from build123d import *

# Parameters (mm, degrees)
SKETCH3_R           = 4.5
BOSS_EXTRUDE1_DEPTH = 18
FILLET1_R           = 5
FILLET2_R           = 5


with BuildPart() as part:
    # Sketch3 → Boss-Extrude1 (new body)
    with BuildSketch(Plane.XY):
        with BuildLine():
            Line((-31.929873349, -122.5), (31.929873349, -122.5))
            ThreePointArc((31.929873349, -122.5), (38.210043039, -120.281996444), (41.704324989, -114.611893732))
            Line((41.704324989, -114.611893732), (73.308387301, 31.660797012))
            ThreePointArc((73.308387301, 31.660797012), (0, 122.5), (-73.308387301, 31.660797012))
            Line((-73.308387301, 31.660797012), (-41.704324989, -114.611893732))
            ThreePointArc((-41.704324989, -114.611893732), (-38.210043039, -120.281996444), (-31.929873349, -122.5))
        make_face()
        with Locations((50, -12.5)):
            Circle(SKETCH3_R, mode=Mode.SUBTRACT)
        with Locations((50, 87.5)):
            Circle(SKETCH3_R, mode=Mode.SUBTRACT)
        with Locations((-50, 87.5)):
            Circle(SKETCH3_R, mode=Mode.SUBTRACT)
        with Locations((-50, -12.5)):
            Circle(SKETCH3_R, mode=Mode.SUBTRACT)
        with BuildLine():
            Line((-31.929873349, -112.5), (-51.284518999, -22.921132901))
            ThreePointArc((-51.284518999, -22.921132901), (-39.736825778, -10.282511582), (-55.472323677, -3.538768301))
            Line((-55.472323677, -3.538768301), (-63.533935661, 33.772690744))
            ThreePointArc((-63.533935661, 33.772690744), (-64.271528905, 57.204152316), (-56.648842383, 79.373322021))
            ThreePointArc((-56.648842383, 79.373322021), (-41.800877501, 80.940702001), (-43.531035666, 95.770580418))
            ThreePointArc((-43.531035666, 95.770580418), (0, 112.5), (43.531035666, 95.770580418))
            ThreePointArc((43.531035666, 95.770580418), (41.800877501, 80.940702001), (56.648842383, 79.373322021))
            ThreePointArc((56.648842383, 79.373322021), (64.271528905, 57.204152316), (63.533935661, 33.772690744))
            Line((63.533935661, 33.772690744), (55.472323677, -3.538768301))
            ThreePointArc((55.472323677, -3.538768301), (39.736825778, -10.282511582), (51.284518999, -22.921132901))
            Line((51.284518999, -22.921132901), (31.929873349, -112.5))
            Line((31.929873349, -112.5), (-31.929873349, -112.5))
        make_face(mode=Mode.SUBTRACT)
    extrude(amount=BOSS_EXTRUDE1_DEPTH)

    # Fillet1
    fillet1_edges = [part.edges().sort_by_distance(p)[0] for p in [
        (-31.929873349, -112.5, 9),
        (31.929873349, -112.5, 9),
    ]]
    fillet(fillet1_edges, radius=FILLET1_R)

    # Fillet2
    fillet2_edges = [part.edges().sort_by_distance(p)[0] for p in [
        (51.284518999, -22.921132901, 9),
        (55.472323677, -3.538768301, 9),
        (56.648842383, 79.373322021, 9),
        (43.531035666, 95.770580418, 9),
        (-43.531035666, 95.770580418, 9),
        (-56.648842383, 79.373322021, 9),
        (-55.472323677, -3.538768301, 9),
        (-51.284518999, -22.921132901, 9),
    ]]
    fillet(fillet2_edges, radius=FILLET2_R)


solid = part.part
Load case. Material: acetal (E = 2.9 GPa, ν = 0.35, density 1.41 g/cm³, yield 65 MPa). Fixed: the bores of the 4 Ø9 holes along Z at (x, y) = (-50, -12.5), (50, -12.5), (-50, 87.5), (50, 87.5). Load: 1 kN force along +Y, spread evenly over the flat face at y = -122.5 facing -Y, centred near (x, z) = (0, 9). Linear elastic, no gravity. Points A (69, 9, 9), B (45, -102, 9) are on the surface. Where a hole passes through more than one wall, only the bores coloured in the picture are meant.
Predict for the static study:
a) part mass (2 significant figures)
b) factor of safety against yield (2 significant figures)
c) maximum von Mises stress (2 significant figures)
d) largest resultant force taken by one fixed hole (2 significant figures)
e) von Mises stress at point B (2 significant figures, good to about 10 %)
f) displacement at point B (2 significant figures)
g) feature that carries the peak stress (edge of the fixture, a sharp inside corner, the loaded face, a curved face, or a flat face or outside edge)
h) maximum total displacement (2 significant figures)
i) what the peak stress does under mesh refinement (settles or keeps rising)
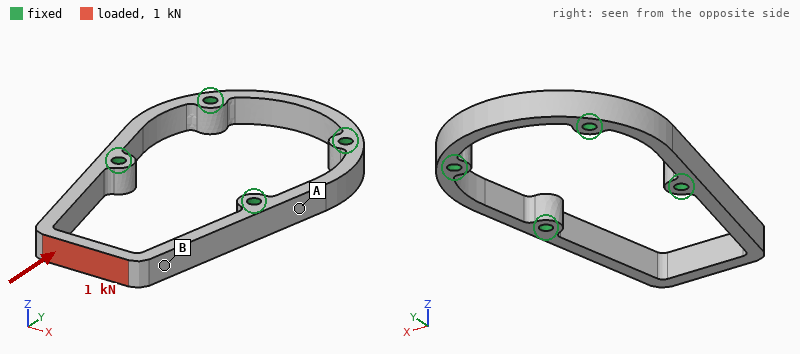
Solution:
180 g
3.3
20 MPa
500 N
7.3 MPa
0.28 mm
the loaded face
0.79 mm
settles
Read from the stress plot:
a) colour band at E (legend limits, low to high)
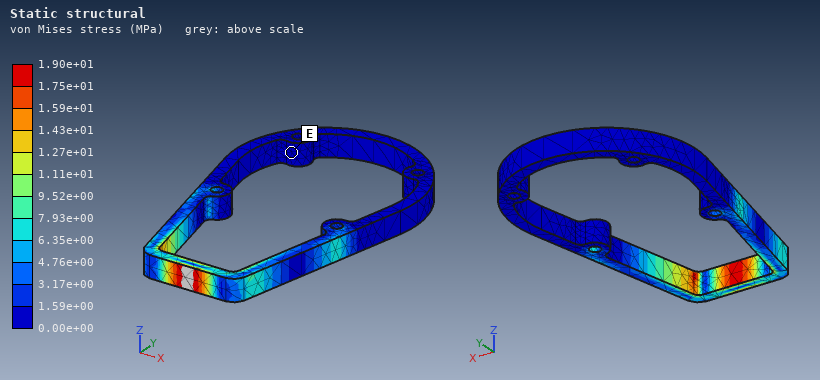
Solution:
0.00e+00 to 1.59e+00 MPa
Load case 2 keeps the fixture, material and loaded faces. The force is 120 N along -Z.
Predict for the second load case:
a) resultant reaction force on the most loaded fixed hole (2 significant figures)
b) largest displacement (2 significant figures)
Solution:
64 N
1.9 mm
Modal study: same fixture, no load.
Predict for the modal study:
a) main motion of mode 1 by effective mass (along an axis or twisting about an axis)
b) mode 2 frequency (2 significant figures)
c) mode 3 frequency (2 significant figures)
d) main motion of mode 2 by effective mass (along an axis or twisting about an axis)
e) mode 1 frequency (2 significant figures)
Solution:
along Z
310 Hz
540 Hz
along X
250 Hz
